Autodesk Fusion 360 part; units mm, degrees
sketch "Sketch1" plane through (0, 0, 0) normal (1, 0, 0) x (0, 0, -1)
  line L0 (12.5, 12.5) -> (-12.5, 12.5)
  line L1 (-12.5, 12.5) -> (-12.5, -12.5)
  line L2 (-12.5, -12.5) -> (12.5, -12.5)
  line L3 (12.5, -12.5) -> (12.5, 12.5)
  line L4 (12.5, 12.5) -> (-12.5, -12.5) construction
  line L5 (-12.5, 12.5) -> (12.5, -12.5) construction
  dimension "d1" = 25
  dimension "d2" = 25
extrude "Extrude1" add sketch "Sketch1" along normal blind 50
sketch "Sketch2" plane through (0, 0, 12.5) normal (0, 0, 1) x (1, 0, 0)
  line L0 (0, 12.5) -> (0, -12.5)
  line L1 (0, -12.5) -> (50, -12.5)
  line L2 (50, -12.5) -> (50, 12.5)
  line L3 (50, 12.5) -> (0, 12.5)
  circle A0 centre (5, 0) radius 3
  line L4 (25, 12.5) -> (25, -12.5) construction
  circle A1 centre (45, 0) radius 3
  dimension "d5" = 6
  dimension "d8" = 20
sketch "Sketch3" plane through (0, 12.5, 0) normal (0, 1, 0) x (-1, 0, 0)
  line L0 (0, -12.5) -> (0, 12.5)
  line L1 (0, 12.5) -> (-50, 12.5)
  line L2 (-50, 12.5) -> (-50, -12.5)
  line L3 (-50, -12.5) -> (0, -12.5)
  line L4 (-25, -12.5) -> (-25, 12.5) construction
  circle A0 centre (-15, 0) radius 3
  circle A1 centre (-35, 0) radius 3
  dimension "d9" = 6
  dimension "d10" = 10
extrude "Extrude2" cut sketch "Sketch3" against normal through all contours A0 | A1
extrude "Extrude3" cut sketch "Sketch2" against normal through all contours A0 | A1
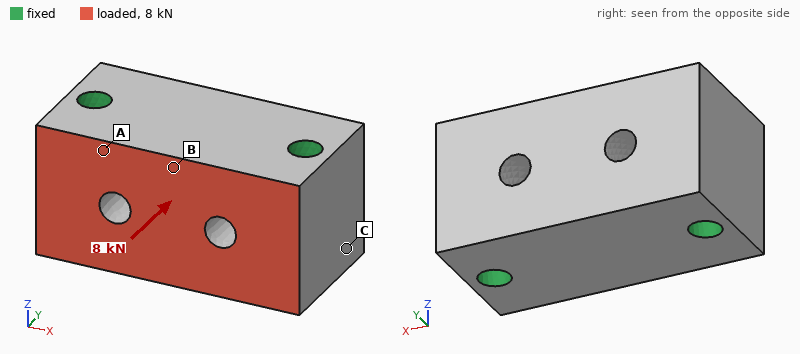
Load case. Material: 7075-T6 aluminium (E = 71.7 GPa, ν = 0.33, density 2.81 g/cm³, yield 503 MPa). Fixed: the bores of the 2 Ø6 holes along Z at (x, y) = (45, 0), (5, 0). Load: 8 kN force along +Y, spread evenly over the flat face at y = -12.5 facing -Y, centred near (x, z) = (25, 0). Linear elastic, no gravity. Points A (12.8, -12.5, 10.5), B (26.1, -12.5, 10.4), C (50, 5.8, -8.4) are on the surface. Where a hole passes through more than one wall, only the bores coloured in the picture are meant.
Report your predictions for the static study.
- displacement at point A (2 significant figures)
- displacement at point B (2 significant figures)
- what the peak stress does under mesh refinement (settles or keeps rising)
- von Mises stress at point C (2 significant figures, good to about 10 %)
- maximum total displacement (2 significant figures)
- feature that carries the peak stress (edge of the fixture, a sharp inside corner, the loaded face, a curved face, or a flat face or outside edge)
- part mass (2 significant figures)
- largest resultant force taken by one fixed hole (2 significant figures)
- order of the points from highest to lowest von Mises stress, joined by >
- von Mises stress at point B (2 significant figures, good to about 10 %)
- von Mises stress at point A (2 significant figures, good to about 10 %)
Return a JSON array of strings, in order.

["3.0 µm", "4.1 µm", "keeps rising", "2.7 MPa", "4.3 µm", "edge of the fixture", "80 g", "4.0 kN", "B > A > C", "10 MPa", "5.8 MPa"]
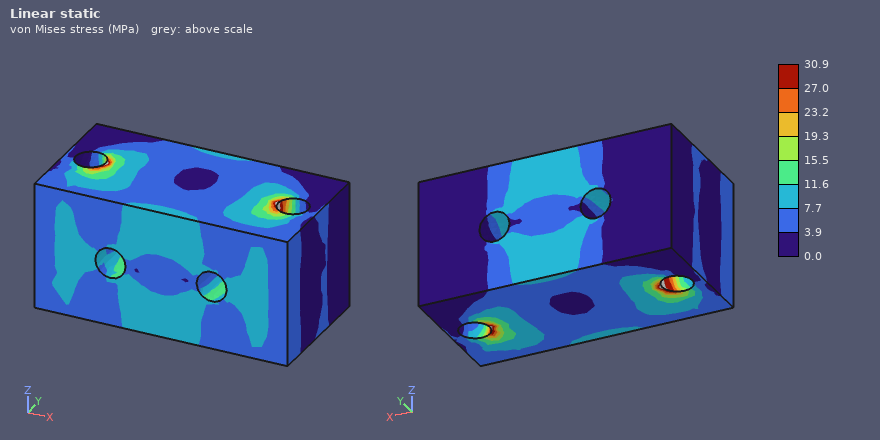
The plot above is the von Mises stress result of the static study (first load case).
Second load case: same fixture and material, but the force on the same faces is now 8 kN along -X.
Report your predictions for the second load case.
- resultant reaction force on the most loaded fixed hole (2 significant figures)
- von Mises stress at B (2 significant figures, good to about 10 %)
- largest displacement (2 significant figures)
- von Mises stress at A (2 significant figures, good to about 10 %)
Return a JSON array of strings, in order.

["4.5 kN", "12 MPa", "6.1 µm", "12 MPa"]
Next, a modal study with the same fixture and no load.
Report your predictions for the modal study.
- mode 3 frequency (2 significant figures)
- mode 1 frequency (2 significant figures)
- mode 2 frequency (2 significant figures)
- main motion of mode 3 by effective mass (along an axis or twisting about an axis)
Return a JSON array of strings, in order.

["32 kHz", "28 kHz", "29 kHz", "twisting about X"]
